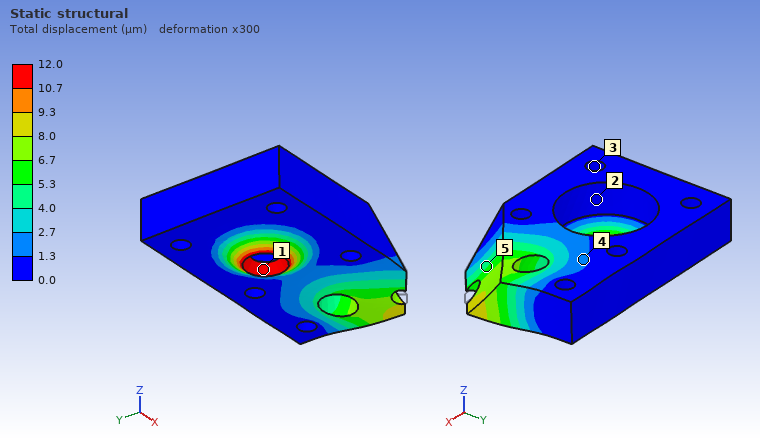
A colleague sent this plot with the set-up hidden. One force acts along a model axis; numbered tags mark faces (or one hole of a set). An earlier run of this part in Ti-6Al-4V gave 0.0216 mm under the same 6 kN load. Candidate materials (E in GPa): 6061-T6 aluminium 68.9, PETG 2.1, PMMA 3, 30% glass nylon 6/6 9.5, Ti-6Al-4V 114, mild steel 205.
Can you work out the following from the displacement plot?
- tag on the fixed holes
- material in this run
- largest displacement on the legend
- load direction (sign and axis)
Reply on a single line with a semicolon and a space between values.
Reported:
3; mild steel; 12.0 µm; -Z
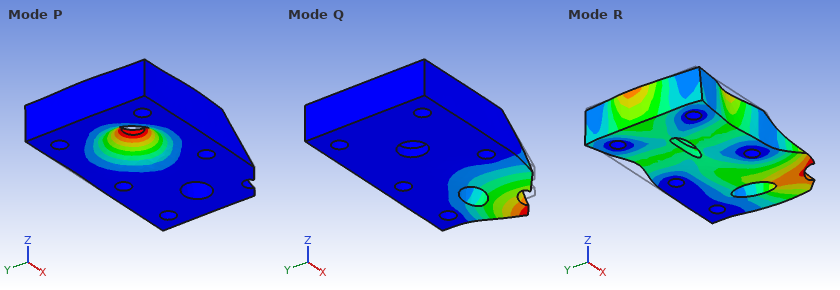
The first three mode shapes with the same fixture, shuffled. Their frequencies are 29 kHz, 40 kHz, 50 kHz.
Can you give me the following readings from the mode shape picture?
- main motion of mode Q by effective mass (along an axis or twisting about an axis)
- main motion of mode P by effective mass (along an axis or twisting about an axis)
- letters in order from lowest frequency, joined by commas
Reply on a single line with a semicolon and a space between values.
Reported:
along Z; along Z; Q, P, R
